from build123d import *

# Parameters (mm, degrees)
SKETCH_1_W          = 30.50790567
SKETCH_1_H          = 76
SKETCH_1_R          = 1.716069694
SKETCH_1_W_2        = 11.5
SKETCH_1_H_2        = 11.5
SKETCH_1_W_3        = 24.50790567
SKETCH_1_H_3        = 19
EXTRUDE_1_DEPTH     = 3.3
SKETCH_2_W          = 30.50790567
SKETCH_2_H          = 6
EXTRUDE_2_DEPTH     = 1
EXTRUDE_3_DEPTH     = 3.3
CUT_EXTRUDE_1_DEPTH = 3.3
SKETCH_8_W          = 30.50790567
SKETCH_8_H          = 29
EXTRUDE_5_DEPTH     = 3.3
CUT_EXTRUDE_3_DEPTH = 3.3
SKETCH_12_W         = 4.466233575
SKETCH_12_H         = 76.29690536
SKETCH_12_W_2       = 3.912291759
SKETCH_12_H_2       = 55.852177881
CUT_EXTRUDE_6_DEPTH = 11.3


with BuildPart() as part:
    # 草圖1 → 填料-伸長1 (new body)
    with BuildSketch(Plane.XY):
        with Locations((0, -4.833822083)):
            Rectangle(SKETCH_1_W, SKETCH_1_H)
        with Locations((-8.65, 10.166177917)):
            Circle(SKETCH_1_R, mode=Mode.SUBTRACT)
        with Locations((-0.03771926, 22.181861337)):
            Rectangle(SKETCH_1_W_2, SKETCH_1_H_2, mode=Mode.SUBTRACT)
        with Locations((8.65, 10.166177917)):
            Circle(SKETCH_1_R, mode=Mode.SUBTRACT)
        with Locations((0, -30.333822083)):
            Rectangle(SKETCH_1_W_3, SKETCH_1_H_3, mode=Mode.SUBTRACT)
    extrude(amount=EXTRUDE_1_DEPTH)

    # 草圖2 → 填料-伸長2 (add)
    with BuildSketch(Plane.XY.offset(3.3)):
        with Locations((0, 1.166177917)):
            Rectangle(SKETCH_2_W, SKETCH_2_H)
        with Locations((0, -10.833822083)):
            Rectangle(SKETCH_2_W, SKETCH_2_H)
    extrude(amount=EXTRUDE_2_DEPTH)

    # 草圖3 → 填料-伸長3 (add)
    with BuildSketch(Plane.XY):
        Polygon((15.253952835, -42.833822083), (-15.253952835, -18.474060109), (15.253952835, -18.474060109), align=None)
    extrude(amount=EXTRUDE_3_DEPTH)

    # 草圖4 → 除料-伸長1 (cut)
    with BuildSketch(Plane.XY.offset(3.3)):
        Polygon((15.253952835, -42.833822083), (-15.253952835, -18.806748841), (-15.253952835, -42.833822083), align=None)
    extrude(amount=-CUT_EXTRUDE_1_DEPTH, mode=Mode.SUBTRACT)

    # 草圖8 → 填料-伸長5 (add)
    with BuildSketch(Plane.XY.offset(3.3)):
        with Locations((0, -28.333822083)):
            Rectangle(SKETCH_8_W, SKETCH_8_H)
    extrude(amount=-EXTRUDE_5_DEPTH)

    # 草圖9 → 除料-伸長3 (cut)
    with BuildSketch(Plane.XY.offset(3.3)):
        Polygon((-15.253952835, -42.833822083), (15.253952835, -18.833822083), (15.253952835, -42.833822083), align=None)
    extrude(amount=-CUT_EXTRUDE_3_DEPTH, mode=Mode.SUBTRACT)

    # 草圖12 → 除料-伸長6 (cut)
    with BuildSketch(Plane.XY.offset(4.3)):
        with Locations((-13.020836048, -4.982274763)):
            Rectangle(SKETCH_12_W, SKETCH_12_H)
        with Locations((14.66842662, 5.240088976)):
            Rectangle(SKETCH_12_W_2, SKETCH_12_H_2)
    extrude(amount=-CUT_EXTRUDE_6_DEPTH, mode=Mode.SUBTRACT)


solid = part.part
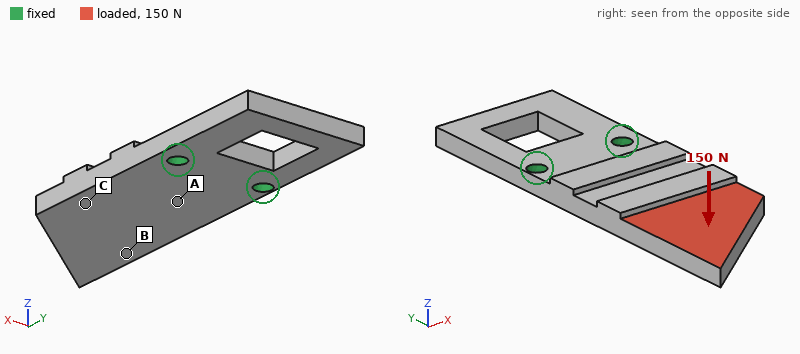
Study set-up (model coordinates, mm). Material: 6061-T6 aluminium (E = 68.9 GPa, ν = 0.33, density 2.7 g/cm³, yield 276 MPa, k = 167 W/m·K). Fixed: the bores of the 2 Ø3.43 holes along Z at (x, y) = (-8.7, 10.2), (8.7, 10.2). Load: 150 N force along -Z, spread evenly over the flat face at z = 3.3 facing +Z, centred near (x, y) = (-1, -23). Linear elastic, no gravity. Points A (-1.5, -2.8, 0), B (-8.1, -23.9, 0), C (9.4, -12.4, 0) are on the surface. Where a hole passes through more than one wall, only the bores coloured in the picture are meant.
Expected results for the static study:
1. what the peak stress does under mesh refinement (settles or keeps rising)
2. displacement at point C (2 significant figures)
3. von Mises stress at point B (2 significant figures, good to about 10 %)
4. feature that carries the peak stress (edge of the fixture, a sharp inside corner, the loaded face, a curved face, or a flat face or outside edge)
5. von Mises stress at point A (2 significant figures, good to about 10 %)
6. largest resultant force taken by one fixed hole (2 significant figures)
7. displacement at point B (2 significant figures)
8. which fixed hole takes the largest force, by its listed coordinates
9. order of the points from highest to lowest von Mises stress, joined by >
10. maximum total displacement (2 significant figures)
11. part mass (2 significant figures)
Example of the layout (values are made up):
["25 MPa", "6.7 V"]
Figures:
["keeps rising", "0.16 mm", "12 MPa", "edge of the fixture", "65 MPa", "82 N", "0.33 mm", "(-8.7, 10.2)", "A > C > B", "0.56 mm", "13 g"]
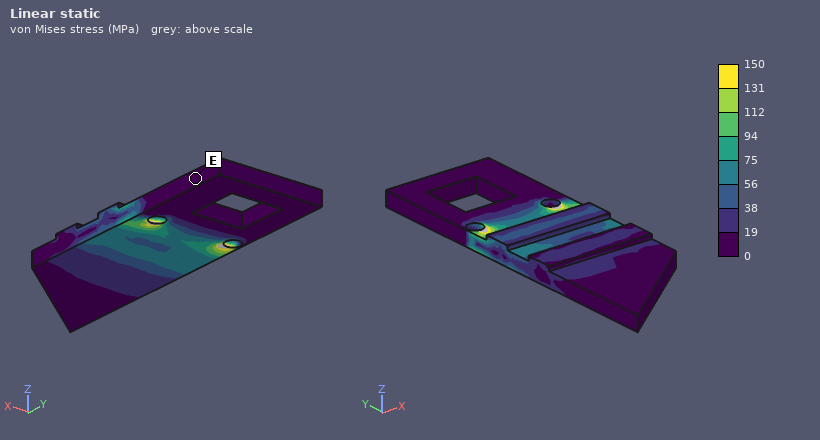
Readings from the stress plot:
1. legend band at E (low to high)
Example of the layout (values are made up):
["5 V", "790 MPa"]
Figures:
["0 to 19 MPa"]
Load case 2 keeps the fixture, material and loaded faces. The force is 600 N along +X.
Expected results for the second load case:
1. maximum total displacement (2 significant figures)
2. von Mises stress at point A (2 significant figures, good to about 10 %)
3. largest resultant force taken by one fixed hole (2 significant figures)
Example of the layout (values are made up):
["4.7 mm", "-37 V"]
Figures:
["77 µm", "8.6 MPa", "1.1 kN"]
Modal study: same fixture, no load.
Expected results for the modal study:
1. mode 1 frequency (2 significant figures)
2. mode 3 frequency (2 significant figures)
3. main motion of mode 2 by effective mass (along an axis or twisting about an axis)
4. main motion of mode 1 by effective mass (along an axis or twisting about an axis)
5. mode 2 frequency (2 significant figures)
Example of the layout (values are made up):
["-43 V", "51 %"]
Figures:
["1700 Hz", "6700 Hz", "along Z", "along Z", "4600 Hz"]
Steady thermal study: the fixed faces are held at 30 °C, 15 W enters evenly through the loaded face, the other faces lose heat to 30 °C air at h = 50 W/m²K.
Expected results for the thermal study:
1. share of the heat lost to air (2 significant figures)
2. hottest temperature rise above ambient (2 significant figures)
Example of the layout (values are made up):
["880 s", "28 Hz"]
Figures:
["12 %", "37 K"]
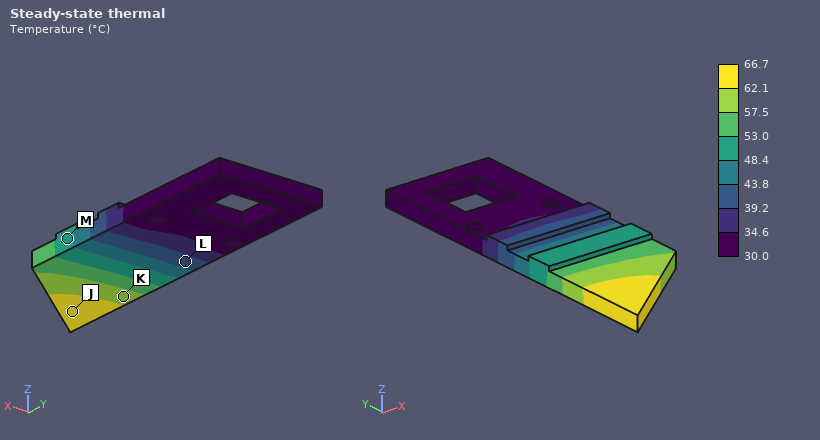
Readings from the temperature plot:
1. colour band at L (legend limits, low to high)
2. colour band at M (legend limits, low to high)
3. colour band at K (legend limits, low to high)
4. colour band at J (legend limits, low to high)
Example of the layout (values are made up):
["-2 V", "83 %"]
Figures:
["39.2 to 43.8 °C", "48.4 to 53.0 °C", "57.5 to 62.1 °C", "62.1 to 66.7 °C"]
